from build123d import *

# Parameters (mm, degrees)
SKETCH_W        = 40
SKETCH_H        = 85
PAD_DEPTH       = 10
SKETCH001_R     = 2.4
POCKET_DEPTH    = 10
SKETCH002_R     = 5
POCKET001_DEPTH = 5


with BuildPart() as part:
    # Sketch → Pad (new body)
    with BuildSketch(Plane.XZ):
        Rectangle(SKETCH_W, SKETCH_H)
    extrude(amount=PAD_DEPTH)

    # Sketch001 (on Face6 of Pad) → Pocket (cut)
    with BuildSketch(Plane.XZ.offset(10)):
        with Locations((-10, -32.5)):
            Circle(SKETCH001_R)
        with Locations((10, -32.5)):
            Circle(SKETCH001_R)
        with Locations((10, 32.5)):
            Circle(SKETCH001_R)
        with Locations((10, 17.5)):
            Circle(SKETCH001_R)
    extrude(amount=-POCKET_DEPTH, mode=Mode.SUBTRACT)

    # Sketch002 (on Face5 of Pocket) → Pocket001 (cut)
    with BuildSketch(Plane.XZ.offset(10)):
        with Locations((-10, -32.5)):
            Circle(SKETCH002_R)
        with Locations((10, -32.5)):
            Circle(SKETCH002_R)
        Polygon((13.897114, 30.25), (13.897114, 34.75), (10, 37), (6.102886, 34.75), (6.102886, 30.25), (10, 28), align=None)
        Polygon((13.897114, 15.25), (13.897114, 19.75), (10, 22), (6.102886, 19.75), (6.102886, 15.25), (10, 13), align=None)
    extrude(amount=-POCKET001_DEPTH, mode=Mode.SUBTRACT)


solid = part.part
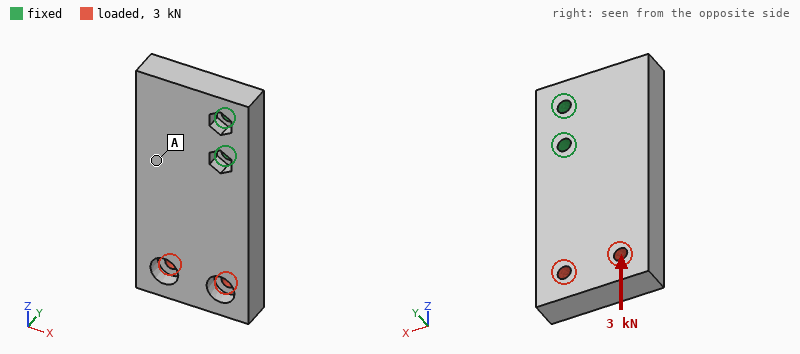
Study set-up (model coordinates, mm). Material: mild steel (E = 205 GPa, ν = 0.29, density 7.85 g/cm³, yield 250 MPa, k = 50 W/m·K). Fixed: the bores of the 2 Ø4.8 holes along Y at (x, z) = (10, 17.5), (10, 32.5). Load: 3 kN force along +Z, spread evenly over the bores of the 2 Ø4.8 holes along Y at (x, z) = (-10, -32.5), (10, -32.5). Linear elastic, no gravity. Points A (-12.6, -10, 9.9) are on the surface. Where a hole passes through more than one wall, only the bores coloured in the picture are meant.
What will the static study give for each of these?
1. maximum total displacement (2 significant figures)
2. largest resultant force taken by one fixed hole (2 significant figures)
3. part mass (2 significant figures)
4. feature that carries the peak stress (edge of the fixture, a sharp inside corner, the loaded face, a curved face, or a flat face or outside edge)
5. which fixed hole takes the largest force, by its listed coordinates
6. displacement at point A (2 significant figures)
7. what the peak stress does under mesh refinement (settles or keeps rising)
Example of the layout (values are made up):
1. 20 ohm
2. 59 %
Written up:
1. 26 µm
2. 2.6 kN
3. 250 g
4. edge of the fixture
5. (10, 17.5)
6. 4.0 µm
7. keeps rising
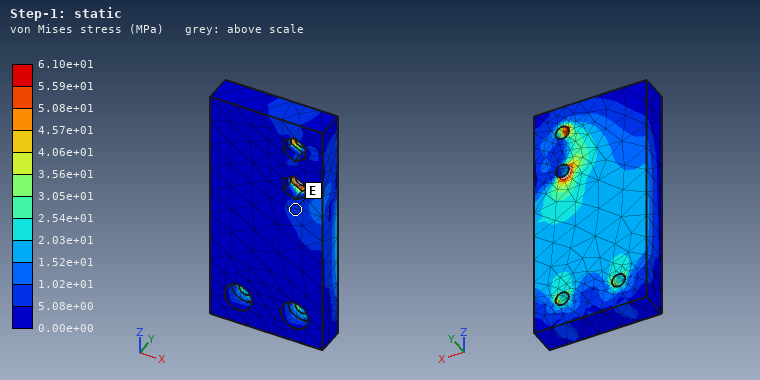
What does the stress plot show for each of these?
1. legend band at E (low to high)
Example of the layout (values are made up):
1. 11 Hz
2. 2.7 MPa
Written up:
1. 5.08e+00 to 1.02e+01 MPa
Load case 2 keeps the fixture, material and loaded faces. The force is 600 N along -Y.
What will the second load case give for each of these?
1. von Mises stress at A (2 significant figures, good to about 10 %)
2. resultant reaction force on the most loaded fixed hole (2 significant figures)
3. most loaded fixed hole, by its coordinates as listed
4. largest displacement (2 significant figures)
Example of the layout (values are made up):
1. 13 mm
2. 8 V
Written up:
1. 32 MPa
2. 2.1 kN
3. (10, 17.5)
4. 86 µm
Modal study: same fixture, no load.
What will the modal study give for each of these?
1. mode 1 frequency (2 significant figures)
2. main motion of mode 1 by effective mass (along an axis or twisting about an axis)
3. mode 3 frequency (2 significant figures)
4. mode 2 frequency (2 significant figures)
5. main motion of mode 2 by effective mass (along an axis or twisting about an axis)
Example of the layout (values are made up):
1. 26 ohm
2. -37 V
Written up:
1. 1700 Hz
2. along Y
3. 3900 Hz
4. 3600 Hz
5. along X
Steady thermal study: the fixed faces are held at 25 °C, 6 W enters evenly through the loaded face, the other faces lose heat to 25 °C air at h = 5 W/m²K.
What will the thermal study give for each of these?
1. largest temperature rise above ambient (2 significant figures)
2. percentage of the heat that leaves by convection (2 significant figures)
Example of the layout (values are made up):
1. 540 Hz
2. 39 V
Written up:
1. 20 K
2. 7.3 %
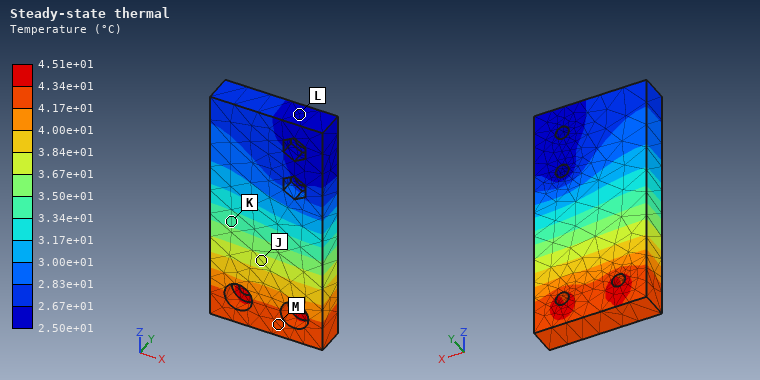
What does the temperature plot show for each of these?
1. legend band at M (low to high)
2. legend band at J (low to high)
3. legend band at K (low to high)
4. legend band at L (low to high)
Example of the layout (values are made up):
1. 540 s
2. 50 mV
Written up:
1. 4.17e+01 to 4.34e+01 °C
2. 3.67e+01 to 3.84e+01 °C
3. 3.34e+01 to 3.50e+01 °C
4. 2.50e+01 to 2.67e+01 °C
